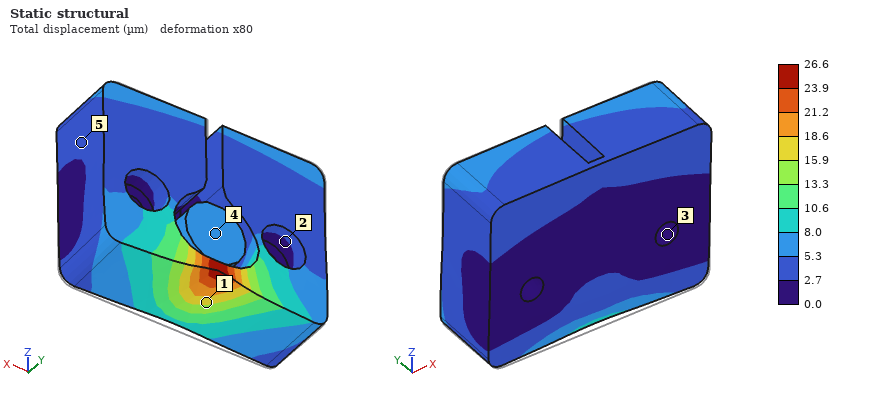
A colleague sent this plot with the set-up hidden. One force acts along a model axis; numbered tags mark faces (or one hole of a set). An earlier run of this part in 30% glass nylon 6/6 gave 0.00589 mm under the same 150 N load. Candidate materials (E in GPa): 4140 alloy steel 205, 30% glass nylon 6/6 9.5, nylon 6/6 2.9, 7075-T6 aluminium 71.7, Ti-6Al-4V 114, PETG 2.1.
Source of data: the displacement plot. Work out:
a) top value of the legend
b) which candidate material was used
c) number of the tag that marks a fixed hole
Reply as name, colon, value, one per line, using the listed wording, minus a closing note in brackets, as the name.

top value of the legend: 26.6 µm
which candidate material was used: PETG
number of the tag that marks a fixed hole: 3
